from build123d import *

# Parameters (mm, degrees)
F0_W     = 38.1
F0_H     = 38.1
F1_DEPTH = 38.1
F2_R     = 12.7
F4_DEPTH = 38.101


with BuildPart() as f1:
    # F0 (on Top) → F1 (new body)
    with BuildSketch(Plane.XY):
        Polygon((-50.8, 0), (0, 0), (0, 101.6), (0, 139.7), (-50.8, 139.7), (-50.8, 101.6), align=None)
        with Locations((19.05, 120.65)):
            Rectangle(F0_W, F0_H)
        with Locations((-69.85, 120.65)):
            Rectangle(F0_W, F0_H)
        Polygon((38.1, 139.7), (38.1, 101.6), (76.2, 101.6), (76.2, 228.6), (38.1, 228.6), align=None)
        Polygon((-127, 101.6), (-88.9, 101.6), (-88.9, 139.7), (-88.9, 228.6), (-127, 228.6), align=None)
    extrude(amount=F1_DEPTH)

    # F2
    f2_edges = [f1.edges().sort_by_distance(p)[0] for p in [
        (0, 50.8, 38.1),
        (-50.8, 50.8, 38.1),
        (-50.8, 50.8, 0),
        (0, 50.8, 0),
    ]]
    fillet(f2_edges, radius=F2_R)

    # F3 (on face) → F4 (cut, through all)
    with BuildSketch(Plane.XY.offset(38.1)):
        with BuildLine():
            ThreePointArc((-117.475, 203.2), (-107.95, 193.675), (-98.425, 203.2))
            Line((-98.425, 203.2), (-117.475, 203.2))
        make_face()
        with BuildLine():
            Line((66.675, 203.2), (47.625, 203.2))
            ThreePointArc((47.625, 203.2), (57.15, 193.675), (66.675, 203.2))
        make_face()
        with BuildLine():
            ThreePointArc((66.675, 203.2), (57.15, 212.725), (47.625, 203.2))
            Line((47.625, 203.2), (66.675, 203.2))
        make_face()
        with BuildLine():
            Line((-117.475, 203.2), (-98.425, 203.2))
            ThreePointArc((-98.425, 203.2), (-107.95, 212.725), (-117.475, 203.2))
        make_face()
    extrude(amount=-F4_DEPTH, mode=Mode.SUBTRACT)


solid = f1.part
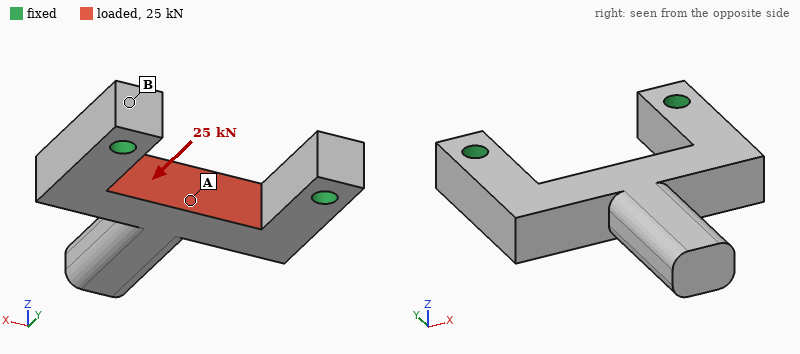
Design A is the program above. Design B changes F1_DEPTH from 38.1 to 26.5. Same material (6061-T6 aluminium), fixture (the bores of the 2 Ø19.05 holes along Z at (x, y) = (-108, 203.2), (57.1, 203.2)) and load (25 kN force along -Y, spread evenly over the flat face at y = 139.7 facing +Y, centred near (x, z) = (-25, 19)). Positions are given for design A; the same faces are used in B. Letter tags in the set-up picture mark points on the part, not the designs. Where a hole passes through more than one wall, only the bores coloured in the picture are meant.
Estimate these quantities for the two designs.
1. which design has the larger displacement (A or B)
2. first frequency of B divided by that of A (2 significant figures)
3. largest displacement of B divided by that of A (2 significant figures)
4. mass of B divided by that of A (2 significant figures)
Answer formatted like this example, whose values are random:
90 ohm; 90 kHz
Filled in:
B; 0.74; 1.4; 0.69
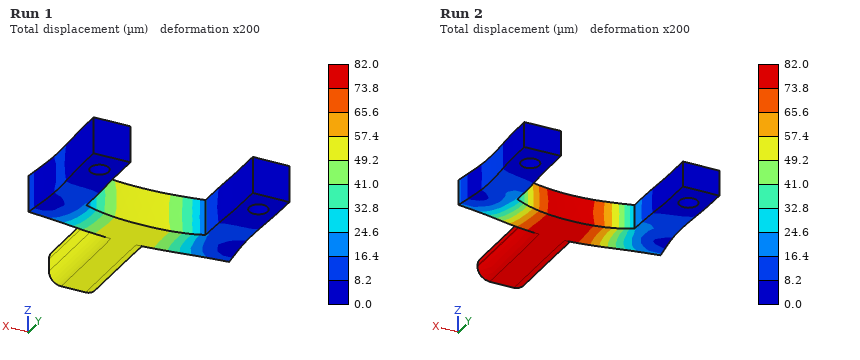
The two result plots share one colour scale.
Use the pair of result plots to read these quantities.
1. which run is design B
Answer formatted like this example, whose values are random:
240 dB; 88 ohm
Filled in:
Run 2
